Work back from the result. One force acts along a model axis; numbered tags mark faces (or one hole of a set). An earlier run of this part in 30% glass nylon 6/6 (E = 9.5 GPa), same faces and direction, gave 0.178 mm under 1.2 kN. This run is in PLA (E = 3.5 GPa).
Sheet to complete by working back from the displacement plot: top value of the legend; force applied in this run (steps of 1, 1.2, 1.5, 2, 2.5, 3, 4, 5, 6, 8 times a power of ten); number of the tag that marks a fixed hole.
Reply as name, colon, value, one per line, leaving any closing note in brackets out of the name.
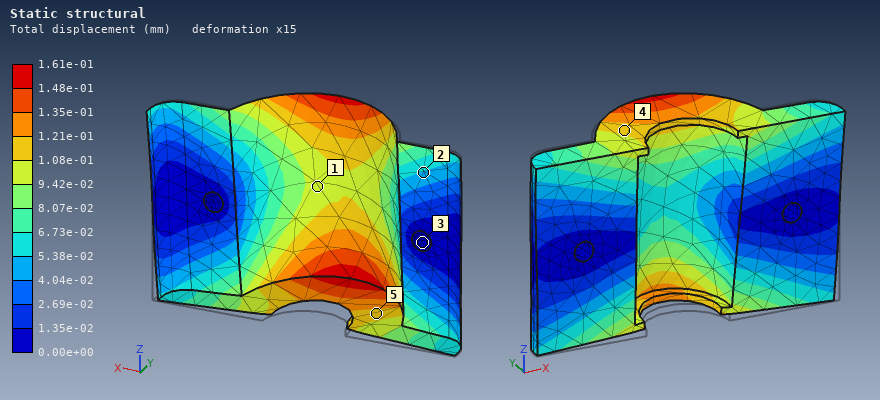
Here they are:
top value of the legend: 1.61e-01 mm
force applied in this run: 400 N
number of the tag that marks a fixed hole: 3
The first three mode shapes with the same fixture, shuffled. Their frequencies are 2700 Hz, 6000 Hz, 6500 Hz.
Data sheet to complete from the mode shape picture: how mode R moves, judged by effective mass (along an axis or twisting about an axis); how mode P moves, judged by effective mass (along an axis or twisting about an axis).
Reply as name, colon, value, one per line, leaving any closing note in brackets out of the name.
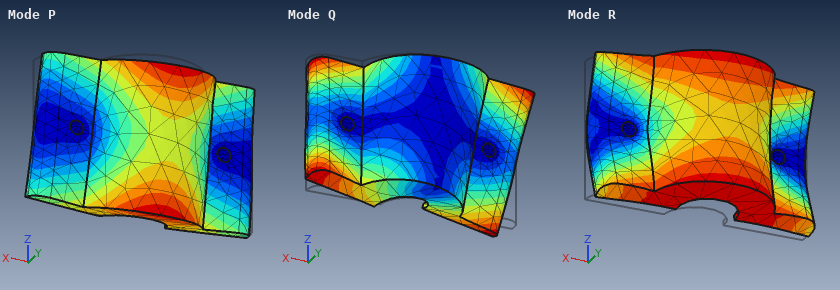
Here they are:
how mode R moves, judged by effective mass: along Y
how mode P moves, judged by effective mass: along Z
